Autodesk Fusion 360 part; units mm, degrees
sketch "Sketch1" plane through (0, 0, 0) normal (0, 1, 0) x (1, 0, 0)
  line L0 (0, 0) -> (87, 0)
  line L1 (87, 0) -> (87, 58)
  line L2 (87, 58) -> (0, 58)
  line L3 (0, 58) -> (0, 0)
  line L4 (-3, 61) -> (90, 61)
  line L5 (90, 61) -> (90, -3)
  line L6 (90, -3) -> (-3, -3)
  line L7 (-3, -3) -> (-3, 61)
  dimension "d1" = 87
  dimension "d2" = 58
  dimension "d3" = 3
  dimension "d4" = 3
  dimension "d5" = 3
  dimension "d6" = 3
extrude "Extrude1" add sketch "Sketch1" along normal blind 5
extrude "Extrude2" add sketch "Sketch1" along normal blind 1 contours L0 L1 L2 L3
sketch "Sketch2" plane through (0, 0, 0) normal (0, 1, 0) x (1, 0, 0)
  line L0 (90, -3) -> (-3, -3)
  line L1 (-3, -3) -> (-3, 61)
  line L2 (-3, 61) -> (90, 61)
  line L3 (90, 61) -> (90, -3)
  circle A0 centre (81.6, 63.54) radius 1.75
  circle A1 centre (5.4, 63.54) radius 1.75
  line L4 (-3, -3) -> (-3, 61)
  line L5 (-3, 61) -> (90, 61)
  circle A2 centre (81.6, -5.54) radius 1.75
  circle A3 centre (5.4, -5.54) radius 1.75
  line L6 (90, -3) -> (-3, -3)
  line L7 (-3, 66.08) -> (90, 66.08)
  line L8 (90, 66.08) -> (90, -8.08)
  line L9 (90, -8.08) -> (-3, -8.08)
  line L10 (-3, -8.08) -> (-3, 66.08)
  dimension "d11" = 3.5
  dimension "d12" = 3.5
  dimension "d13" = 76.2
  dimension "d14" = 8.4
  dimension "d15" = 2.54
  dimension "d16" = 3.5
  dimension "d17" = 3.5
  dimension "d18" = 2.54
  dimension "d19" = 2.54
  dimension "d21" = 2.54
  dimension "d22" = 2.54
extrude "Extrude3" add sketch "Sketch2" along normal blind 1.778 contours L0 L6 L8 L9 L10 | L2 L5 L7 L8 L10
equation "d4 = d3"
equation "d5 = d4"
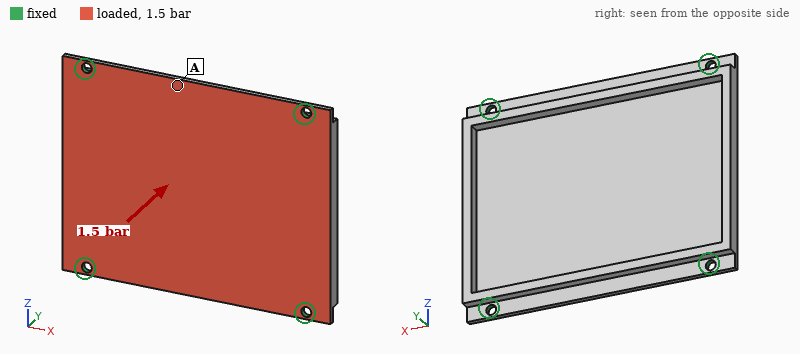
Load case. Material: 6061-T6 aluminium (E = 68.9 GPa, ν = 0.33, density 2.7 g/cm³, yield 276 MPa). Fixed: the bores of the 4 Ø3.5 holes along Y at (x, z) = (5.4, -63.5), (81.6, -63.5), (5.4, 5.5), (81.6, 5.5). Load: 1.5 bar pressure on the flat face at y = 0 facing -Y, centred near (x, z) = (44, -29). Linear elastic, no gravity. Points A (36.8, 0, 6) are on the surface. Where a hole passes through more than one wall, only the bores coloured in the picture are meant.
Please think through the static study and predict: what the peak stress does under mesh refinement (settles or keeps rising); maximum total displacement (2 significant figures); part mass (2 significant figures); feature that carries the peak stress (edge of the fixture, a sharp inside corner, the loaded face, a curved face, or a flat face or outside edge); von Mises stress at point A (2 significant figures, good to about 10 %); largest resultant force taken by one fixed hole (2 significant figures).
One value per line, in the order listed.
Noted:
keeps rising
1.2 mm
30 g
edge of the fixture
30 MPa
270 N
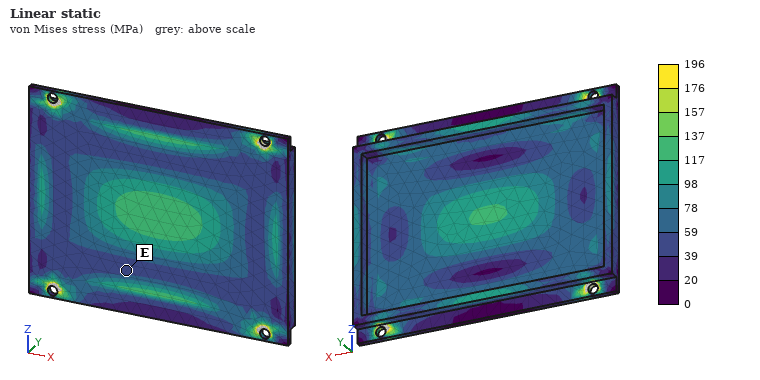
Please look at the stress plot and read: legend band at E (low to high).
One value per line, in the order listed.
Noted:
39 to 59 MPa
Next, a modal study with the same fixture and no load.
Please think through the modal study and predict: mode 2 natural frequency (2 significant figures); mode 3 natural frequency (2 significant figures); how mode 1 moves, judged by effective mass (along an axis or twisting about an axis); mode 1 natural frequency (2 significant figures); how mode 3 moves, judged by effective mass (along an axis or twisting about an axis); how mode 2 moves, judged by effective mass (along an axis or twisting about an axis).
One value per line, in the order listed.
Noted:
2400 Hz
2700 Hz
along Y
1400 Hz
twisting about X
twisting about Z
